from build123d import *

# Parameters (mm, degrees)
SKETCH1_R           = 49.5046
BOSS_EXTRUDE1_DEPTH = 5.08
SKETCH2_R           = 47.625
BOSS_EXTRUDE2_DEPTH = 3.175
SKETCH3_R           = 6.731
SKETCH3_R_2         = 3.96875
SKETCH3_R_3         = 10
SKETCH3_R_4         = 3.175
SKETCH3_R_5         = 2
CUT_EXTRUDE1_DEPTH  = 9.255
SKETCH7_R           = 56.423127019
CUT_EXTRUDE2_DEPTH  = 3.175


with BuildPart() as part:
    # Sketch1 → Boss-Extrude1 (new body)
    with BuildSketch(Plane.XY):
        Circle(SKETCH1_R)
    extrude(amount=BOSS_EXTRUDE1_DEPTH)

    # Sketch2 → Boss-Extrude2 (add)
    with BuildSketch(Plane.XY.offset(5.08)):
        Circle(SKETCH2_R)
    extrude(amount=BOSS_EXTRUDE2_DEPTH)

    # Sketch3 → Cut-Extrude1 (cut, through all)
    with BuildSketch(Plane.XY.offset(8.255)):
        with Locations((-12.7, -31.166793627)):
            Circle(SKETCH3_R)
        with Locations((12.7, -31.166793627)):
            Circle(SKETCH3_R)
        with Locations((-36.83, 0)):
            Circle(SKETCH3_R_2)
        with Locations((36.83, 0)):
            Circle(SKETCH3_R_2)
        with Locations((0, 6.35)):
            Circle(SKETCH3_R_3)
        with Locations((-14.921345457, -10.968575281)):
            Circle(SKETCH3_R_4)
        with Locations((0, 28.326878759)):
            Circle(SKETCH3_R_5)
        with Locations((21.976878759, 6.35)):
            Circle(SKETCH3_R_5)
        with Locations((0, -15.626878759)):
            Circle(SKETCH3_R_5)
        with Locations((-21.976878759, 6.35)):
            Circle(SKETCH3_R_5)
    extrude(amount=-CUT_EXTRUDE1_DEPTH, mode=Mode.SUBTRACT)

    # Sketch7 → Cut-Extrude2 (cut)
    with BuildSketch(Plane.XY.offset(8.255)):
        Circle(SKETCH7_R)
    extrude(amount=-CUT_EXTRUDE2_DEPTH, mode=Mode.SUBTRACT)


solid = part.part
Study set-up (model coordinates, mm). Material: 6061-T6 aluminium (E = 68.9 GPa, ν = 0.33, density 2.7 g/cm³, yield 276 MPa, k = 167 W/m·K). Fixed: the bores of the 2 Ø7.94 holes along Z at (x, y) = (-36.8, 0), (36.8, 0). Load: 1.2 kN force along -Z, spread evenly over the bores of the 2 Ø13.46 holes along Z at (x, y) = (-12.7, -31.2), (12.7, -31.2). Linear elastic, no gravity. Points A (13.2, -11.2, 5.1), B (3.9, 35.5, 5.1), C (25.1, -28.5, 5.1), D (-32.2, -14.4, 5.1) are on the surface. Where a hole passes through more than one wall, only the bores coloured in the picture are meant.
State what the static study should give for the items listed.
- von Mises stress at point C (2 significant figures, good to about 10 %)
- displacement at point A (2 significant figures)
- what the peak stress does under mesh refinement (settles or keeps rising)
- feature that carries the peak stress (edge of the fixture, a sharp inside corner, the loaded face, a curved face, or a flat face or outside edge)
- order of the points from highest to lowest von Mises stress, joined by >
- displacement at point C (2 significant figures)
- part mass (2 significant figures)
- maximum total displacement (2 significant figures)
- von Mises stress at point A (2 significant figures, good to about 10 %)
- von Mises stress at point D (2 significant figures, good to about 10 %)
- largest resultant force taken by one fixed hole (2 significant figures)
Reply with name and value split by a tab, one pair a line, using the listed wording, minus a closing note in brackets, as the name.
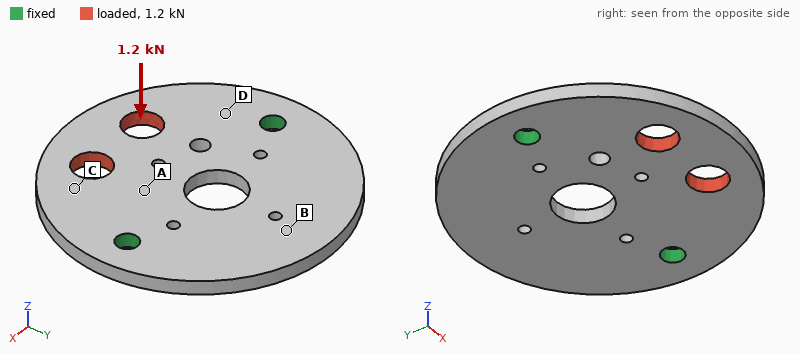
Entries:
von Mises stress at point C	30 MPa
displacement at point A	0.11 mm
what the peak stress does under mesh refinement	keeps rising
feature that carries the peak stress	edge of the fixture
order of the points from highest to lowest von Mises stress, joined by >	D > A > C > B
displacement at point C	0.23 mm
part mass	95 g
maximum total displacement	0.56 mm
von Mises stress at point A	55 MPa
von Mises stress at point D	70 MPa
largest resultant force taken by one fixed hole	600 N
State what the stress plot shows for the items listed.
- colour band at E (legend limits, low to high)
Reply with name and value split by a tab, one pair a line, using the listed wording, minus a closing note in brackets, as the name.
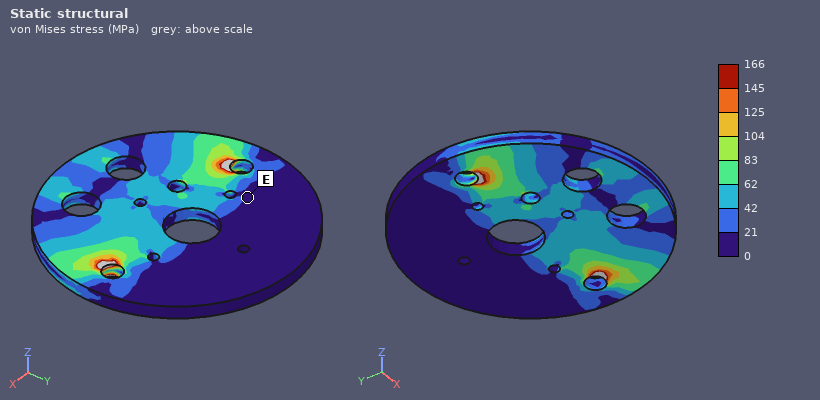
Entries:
colour band at E	0 to 21 MPa
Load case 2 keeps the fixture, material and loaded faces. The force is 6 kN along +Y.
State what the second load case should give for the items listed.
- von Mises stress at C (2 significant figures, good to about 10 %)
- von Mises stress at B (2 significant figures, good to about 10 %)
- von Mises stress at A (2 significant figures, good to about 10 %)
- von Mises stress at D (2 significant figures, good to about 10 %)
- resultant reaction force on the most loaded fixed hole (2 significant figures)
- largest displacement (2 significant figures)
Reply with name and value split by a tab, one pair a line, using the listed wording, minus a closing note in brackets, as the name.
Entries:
von Mises stress at C	22 MPa
von Mises stress at B	4.6 MPa
von Mises stress at A	19 MPa
von Mises stress at D	21 MPa
resultant reaction force on the most loaded fixed hole	3.1 kN
largest displacement	21 µm
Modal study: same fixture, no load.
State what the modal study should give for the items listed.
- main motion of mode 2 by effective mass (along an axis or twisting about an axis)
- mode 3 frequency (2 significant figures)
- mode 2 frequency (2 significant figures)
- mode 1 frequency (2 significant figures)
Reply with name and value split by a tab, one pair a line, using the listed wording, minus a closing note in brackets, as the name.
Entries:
main motion of mode 2 by effective mass	along Z
mode 3 frequency	4400 Hz
mode 2 frequency	2100 Hz
mode 1 frequency	1700 Hz
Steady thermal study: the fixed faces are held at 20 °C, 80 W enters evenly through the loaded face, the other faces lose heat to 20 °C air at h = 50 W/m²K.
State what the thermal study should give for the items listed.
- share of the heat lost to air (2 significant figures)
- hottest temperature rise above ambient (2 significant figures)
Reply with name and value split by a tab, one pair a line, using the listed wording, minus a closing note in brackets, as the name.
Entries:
share of the heat lost to air	17 %
hottest temperature rise above ambient	56 K
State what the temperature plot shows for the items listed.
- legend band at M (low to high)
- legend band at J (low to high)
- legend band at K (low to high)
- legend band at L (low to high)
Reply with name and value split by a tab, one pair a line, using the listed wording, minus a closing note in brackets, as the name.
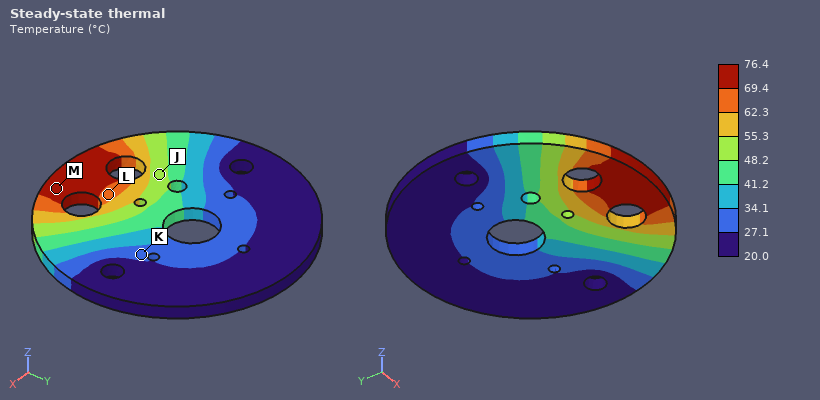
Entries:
legend band at M	69.4 to 76.4 °C
legend band at J	48.2 to 55.3 °C
legend band at K	27.1 to 34.1 °C
legend band at L	62.3 to 69.4 °C
